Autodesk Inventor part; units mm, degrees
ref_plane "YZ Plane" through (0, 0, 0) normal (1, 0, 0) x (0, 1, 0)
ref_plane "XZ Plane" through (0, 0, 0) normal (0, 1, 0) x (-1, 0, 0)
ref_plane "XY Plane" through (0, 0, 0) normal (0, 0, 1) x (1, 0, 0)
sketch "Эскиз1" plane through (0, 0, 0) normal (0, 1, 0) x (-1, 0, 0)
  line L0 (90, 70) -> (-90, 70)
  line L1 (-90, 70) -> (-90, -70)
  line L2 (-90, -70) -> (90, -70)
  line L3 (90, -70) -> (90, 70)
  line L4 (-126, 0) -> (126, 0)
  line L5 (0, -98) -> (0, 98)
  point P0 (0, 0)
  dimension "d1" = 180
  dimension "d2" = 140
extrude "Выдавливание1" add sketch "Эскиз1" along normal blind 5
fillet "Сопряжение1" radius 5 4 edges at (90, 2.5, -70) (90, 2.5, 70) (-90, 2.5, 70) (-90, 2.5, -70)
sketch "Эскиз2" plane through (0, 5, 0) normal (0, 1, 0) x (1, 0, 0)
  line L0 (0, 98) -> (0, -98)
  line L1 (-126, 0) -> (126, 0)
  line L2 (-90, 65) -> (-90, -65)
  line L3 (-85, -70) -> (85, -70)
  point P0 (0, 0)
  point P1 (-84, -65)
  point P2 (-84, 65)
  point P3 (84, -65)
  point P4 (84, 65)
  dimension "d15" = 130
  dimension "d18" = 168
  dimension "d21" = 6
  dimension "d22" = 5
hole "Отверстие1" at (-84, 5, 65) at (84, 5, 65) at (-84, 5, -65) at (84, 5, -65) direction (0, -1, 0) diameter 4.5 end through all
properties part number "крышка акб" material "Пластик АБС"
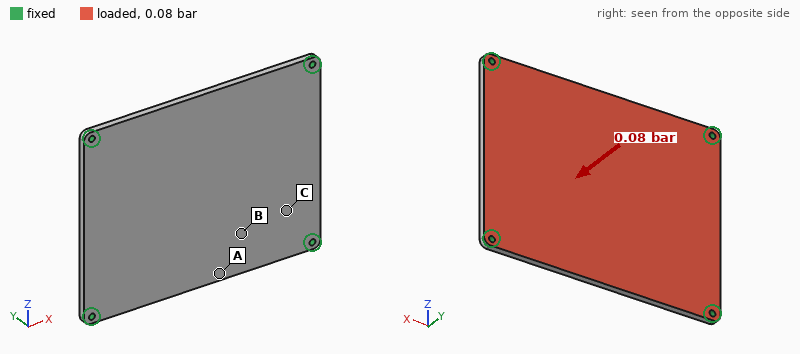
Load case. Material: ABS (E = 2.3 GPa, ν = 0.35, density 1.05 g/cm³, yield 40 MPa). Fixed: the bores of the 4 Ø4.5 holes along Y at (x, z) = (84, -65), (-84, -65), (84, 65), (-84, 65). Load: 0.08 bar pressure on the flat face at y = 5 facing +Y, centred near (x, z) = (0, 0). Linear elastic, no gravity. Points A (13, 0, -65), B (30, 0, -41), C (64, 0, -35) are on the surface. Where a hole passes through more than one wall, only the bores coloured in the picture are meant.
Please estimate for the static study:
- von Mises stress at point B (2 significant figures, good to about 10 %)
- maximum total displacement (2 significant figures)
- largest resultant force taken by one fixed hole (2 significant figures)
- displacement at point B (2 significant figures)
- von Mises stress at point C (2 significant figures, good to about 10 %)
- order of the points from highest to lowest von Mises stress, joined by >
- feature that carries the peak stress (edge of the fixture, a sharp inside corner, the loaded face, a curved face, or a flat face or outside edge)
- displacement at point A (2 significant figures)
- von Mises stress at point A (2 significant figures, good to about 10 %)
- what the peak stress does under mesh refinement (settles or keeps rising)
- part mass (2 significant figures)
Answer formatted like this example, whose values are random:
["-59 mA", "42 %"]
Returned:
["2.4 MPa", "1.5 mm", "50 N", "1.2 mm", "1.2 MPa", "A > B > C", "edge of the fixture", "1.2 mm", "3.5 MPa", "keeps rising", "130 g"]
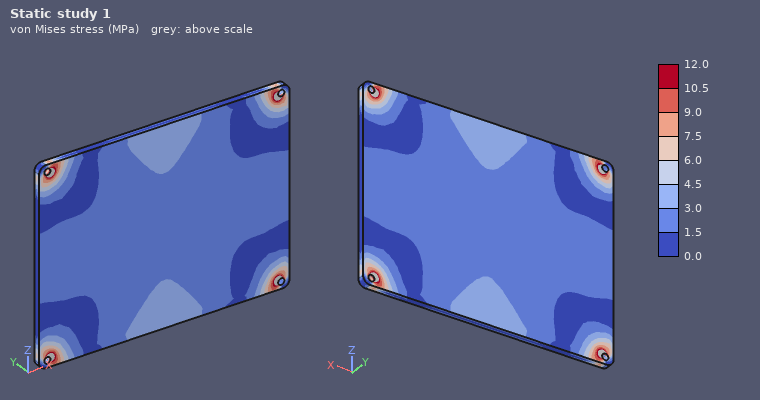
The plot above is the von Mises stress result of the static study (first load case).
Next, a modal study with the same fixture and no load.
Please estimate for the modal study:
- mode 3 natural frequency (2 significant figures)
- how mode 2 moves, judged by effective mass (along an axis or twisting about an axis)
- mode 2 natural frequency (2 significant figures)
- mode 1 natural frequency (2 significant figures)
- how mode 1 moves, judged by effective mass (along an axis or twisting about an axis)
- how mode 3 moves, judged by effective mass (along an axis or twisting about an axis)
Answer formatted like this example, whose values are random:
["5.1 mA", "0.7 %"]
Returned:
["410 Hz", "twisting about X", "320 Hz", "180 Hz", "along Y", "twisting about Z"]
